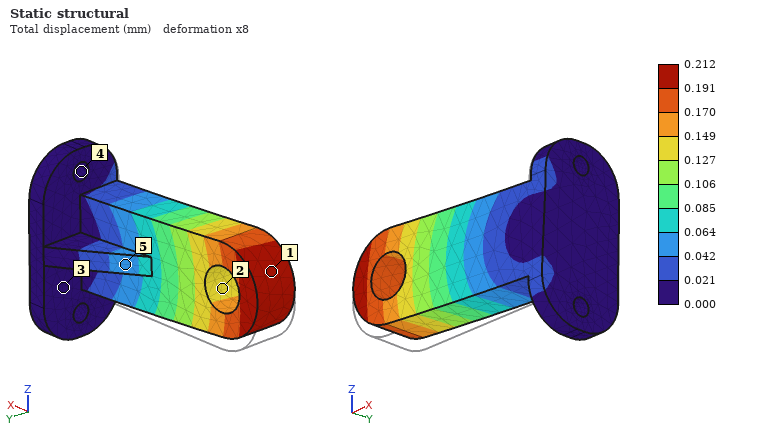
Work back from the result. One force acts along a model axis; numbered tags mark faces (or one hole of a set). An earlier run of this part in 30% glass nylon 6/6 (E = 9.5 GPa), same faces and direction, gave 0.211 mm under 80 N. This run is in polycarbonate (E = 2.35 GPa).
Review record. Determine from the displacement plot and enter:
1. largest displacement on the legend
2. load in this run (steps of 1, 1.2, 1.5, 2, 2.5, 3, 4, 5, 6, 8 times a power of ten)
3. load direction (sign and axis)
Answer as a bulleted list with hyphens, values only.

- 0.212 mm
- 20 N
- +Z
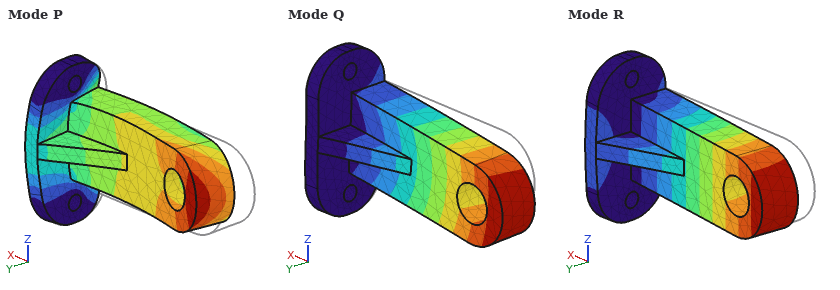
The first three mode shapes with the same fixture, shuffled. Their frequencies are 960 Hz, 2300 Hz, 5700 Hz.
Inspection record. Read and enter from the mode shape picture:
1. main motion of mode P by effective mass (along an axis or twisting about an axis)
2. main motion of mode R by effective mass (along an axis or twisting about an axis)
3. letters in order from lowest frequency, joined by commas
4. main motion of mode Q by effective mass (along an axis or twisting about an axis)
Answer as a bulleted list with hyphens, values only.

- along X
- along Y
- R, Q, P
- along Z
